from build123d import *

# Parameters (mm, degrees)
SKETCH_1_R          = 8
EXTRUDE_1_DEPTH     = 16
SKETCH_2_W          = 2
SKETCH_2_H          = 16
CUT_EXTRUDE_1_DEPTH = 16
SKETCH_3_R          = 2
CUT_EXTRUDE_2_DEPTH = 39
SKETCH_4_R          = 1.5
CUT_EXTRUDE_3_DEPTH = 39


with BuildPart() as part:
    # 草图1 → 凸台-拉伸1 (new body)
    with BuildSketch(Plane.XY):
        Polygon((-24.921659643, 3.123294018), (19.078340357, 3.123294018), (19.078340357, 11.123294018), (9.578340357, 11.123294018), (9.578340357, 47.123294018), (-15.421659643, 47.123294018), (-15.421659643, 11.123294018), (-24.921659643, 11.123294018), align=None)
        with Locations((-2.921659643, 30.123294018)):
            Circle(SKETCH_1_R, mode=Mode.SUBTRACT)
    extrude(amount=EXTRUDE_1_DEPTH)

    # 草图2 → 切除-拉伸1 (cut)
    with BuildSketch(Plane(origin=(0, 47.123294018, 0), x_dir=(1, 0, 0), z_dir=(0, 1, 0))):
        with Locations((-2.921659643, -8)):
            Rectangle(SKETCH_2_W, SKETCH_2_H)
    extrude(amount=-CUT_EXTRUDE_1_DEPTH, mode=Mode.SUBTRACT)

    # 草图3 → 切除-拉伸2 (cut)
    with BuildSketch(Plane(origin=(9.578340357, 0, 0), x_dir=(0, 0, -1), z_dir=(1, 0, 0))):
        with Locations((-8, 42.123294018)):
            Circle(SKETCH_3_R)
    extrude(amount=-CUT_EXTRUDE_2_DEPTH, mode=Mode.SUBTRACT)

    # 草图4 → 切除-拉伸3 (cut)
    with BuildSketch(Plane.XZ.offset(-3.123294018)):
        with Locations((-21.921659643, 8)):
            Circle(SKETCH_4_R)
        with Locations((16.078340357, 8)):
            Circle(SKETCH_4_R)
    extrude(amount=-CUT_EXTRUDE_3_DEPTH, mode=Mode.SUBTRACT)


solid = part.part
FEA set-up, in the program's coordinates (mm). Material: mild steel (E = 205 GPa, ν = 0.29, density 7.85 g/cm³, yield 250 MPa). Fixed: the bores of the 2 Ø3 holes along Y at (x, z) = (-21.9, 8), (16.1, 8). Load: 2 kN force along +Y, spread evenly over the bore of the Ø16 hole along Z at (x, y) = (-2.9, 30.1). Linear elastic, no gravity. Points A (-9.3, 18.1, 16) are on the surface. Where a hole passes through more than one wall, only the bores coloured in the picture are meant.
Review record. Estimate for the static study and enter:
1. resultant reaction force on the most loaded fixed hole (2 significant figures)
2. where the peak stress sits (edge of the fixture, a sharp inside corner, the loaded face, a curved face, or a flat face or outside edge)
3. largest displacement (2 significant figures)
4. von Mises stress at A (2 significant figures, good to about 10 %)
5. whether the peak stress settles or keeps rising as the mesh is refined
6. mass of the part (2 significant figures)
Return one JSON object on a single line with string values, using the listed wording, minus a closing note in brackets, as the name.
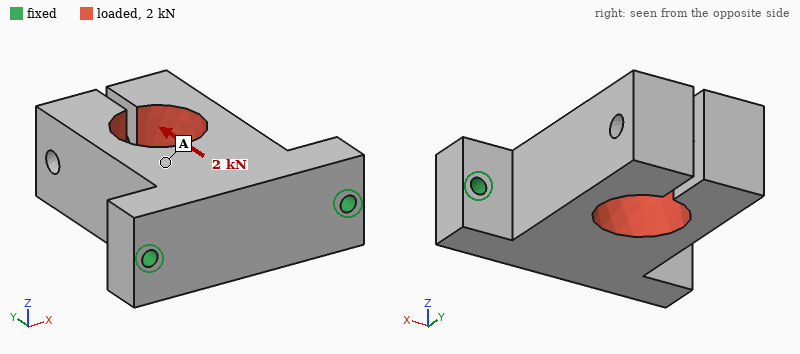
{"resultant reaction force on the most loaded fixed hole": "1.1 kN", "where the peak stress sits": "edge of the fixture", "largest displacement": "19 µm", "von Mises stress at A": "9.1 MPa", "whether the peak stress settles or keeps rising as the mesh is refined": "keeps rising", "mass of the part": "130 g"}
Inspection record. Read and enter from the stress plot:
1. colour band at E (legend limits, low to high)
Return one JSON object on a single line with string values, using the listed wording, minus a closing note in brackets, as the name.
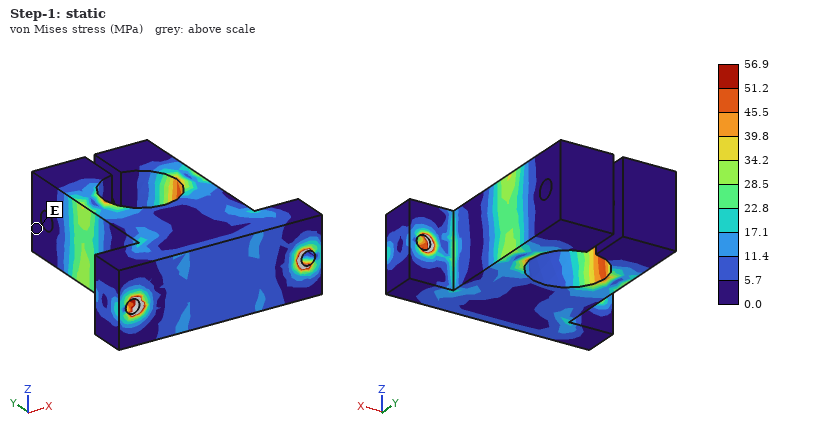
{"colour band at E": "0.0 to 5.7 MPa"}
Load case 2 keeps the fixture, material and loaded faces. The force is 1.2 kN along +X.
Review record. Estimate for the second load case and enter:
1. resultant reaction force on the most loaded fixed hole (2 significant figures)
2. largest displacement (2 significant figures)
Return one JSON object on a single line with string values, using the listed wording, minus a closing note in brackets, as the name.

{"resultant reaction force on the most loaded fixed hole": "1.0 kN", "largest displacement": "22 µm"}
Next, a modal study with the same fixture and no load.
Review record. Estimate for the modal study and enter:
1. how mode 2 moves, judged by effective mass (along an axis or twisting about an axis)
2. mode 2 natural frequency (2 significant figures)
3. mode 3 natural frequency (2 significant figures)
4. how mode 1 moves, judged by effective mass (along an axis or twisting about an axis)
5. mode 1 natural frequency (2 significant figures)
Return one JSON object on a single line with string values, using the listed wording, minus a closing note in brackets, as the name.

{"how mode 2 moves, judged by effective mass": "along X", "mode 2 natural frequency": "4300 Hz", "mode 3 natural frequency": "4500 Hz", "how mode 1 moves, judged by effective mass": "along Z", "mode 1 natural frequency": "3500 Hz"}
